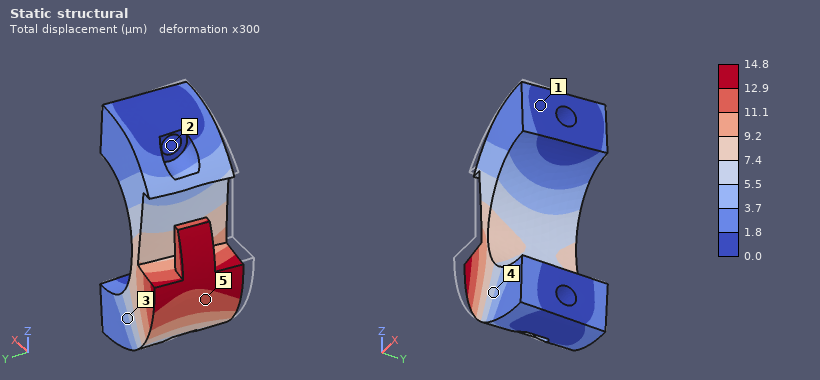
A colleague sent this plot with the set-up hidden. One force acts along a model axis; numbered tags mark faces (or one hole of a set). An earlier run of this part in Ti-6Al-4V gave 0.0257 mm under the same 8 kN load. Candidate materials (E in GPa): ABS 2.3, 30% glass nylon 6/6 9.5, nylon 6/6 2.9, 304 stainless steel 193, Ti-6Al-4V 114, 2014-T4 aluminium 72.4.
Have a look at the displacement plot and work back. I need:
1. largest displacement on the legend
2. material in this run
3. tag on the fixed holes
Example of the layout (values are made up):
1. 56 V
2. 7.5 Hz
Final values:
1. 14.8 µm
2. 304 stainless steel
3. 2
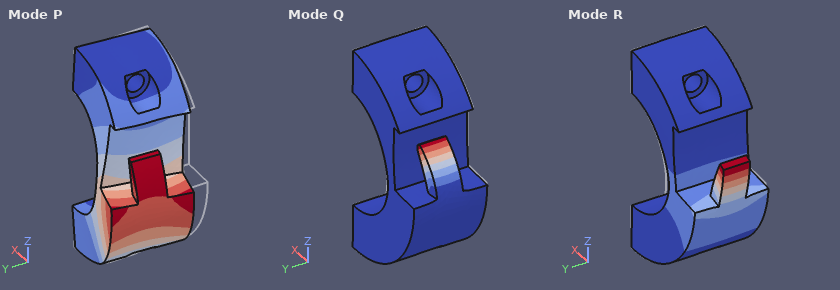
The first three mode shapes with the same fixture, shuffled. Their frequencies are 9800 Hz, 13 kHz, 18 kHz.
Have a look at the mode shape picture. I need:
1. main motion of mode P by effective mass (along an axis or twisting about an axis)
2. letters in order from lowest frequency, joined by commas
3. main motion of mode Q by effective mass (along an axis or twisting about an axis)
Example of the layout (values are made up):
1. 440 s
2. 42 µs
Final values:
1. along Y
2. P, R, Q
3. along Z
